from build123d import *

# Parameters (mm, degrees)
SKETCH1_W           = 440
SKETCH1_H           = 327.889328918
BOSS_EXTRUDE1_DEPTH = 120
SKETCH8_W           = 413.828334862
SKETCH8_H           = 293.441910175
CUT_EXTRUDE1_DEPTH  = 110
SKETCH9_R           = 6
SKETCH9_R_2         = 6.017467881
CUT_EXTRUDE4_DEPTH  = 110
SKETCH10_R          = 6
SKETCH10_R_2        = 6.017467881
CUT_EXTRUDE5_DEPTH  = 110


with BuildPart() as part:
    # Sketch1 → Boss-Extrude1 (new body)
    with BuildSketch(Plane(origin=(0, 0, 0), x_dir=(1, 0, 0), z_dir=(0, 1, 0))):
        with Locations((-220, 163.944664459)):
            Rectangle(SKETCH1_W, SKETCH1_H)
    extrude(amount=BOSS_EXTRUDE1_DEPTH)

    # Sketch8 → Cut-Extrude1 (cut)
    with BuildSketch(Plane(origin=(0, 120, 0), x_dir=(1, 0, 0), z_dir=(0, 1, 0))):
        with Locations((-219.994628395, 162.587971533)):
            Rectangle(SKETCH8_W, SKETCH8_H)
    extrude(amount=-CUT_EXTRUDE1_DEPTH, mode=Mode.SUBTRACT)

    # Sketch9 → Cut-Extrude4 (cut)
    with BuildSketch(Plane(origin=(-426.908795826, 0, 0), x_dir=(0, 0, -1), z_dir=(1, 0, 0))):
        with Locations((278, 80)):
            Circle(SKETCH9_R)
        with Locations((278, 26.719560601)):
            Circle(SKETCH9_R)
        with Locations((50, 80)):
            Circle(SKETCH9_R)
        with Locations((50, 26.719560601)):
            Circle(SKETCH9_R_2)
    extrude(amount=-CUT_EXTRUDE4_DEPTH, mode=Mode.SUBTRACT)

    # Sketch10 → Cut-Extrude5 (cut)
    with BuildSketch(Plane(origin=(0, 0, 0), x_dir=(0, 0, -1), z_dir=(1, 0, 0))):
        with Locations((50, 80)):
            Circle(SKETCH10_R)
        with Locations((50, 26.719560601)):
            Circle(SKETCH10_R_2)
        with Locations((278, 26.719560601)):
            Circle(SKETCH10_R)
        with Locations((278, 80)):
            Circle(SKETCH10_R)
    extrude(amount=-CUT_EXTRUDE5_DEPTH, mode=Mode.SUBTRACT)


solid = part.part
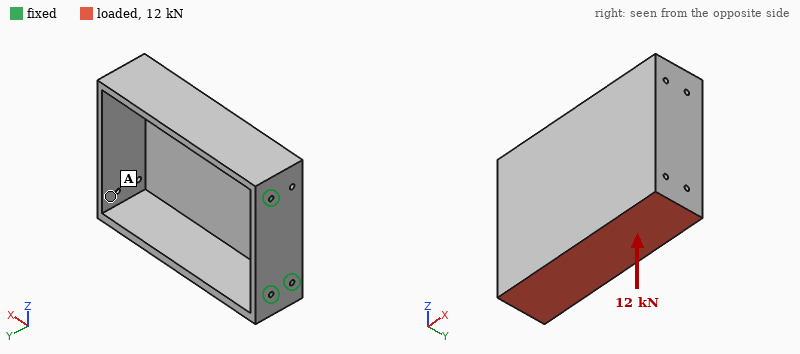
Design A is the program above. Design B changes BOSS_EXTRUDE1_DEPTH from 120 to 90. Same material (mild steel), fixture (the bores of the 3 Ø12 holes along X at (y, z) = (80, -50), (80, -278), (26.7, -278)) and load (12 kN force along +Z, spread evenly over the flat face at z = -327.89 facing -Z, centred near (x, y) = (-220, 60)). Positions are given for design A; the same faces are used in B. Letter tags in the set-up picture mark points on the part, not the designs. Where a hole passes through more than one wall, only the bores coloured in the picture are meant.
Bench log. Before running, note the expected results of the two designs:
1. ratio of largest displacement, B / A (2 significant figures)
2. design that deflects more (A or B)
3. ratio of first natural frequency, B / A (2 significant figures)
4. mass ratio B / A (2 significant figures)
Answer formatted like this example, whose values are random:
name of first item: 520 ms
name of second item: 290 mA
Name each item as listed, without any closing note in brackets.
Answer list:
ratio of largest displacement, B / A: 1.2
design that deflects more: B
ratio of first natural frequency, B / A: 0.92
mass ratio B / A: 0.83
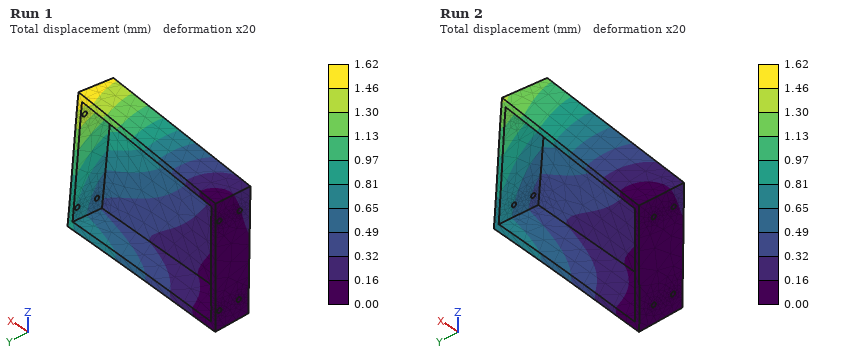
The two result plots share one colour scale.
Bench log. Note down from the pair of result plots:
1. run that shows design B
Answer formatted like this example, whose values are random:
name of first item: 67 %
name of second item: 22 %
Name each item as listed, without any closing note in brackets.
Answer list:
run that shows design B: Run 1
